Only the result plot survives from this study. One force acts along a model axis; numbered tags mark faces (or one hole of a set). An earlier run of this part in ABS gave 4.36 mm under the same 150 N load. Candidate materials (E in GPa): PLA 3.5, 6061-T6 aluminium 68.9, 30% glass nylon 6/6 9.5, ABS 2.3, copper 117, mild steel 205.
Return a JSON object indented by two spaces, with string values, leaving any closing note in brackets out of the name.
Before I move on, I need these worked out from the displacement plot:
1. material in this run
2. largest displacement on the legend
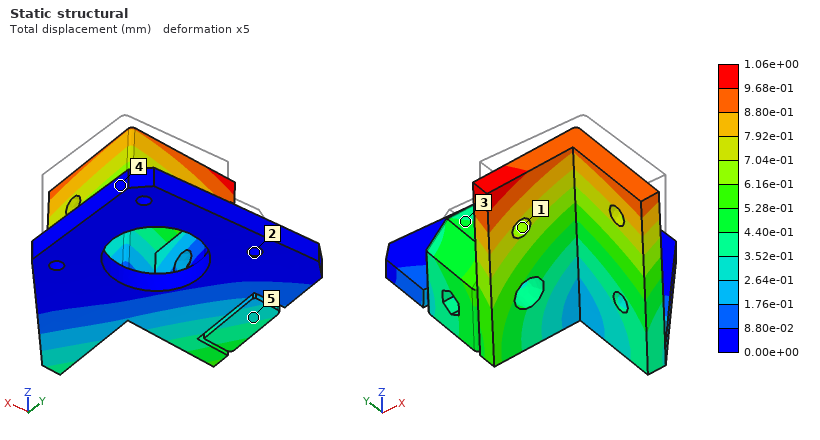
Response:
{
  "material in this run": "30% glass nylon 6/6",
  "largest displacement on the legend": "1.06e+00 mm"
}
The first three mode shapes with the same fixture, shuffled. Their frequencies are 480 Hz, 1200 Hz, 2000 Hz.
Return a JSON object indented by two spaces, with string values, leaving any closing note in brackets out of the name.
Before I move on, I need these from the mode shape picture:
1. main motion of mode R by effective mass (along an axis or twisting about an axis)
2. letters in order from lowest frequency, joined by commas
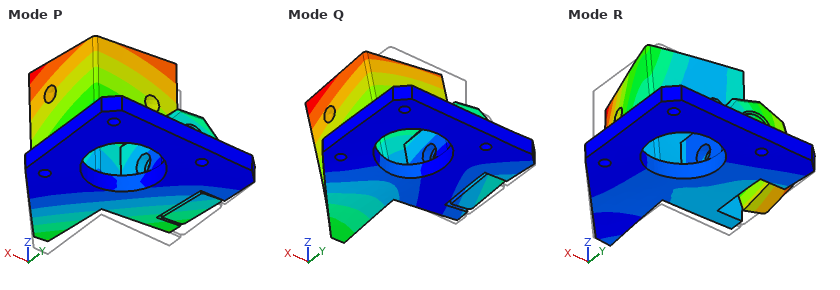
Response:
{
  "main motion of mode R by effective mass": "along Z",
  "letters in order from lowest frequency, joined by commas": "P, Q, R"
}
